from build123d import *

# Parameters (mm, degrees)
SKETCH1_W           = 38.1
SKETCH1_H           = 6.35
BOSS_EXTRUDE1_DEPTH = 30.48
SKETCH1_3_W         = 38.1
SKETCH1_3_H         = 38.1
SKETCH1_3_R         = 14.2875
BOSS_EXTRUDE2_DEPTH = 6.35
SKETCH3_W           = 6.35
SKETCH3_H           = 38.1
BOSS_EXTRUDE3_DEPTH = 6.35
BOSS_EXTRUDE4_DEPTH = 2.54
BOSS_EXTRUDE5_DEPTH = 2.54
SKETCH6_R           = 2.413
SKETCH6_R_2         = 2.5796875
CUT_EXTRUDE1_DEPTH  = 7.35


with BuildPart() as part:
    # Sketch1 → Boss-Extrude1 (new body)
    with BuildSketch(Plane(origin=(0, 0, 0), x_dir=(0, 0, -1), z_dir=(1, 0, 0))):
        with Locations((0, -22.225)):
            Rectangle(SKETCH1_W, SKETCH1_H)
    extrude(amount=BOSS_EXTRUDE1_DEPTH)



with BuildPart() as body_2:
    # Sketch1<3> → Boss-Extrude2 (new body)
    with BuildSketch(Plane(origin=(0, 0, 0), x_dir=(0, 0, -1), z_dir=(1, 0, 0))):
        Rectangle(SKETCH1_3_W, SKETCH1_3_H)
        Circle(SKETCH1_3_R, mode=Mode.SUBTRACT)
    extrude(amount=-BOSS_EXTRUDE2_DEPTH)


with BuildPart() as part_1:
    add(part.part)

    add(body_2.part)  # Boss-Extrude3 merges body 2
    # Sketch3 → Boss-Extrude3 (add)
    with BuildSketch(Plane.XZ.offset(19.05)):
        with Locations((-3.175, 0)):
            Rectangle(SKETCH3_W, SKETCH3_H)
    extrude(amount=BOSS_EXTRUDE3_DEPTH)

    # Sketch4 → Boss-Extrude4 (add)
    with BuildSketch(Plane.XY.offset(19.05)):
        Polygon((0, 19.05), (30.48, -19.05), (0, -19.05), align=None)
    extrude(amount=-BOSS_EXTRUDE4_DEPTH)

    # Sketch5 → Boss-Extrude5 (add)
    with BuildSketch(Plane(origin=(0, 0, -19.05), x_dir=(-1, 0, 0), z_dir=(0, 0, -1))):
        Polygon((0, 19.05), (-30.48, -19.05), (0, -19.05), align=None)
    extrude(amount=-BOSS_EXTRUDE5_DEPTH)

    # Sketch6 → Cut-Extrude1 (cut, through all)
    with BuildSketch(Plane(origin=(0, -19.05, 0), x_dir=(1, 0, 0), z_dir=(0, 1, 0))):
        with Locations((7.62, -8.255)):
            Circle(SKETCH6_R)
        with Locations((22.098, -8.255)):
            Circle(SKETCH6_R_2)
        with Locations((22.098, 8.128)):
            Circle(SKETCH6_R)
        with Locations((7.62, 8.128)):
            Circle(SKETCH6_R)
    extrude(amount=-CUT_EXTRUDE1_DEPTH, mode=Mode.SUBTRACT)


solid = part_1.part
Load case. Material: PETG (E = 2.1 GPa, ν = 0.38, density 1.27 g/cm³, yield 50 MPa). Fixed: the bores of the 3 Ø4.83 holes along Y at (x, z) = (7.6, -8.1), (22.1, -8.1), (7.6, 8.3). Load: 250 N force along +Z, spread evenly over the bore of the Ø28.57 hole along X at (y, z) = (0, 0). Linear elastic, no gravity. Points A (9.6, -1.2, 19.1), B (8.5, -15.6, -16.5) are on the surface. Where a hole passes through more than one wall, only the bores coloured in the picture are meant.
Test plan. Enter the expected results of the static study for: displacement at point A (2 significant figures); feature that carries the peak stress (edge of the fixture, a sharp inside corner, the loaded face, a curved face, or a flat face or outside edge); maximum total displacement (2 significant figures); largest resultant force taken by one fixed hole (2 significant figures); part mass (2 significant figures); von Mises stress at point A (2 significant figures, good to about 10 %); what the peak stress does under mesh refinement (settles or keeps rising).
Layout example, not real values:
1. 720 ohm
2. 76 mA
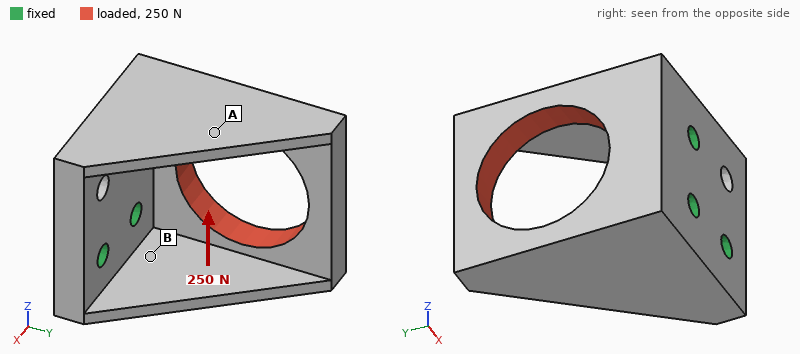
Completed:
1. 0.35 mm
2. edge of the fixture
3. 0.74 mm
4. 280 N
5. 21 g
6. 3.1 MPa
7. keeps rising
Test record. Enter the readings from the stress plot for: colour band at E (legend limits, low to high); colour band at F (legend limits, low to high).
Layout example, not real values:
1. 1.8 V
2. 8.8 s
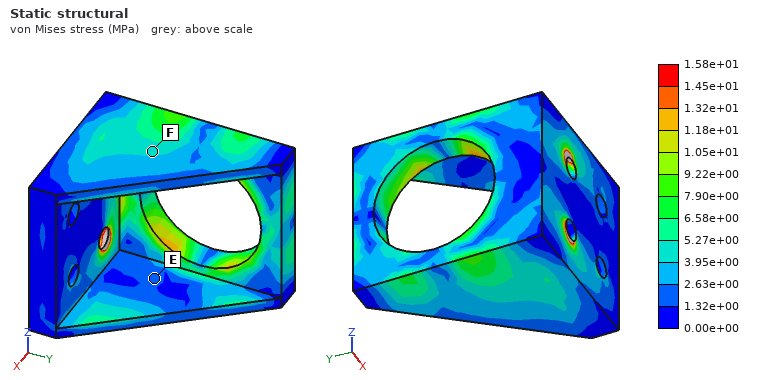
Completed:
1. 1.32e+00 to 2.63e+00 MPa
2. 3.95e+00 to 5.27e+00 MPa
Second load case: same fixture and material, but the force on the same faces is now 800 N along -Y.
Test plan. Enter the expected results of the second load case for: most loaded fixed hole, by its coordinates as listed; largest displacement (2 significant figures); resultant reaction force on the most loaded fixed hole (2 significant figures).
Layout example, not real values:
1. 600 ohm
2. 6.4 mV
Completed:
1. (7.6, -8.1)
2. 0.82 mm
3. 530 N
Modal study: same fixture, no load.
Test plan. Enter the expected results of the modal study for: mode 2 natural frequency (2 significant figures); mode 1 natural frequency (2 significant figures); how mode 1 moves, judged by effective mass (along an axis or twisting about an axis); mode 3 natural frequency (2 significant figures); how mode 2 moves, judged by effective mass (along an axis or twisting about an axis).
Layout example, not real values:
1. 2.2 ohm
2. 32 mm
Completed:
1. 1300 Hz
2. 1100 Hz
3. along Z
4. 2300 Hz
5. along X
